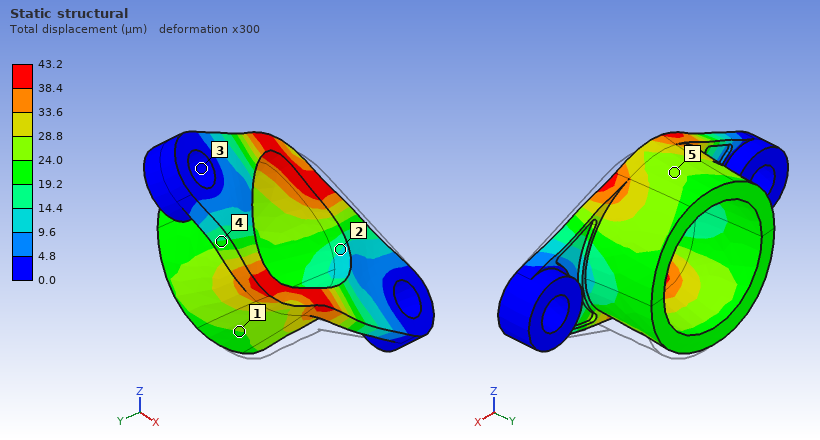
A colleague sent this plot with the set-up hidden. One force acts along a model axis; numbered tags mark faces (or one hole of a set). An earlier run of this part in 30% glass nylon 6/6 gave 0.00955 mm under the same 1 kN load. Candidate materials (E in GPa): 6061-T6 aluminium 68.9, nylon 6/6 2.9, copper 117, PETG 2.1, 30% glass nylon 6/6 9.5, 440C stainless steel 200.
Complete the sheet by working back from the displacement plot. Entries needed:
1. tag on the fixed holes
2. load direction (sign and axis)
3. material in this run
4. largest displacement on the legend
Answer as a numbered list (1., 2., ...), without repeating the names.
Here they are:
1. 3
2. -X
3. PETG
4. 43.2 µm
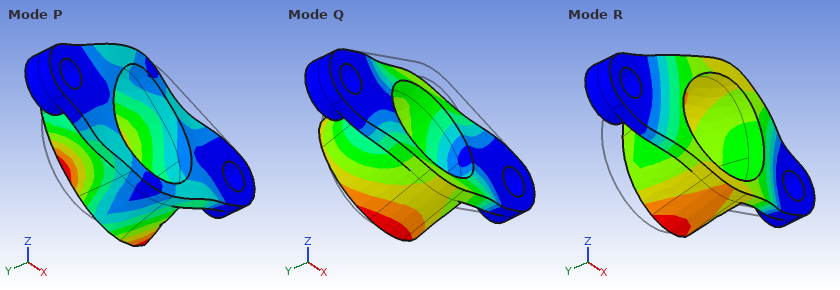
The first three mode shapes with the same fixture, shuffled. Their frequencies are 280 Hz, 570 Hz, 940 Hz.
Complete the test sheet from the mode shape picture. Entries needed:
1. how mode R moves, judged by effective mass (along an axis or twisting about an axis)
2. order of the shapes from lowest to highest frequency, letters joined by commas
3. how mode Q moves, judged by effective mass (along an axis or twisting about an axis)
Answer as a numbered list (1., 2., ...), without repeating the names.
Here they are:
1. along Y
2. Q, R, P
3. along Z
